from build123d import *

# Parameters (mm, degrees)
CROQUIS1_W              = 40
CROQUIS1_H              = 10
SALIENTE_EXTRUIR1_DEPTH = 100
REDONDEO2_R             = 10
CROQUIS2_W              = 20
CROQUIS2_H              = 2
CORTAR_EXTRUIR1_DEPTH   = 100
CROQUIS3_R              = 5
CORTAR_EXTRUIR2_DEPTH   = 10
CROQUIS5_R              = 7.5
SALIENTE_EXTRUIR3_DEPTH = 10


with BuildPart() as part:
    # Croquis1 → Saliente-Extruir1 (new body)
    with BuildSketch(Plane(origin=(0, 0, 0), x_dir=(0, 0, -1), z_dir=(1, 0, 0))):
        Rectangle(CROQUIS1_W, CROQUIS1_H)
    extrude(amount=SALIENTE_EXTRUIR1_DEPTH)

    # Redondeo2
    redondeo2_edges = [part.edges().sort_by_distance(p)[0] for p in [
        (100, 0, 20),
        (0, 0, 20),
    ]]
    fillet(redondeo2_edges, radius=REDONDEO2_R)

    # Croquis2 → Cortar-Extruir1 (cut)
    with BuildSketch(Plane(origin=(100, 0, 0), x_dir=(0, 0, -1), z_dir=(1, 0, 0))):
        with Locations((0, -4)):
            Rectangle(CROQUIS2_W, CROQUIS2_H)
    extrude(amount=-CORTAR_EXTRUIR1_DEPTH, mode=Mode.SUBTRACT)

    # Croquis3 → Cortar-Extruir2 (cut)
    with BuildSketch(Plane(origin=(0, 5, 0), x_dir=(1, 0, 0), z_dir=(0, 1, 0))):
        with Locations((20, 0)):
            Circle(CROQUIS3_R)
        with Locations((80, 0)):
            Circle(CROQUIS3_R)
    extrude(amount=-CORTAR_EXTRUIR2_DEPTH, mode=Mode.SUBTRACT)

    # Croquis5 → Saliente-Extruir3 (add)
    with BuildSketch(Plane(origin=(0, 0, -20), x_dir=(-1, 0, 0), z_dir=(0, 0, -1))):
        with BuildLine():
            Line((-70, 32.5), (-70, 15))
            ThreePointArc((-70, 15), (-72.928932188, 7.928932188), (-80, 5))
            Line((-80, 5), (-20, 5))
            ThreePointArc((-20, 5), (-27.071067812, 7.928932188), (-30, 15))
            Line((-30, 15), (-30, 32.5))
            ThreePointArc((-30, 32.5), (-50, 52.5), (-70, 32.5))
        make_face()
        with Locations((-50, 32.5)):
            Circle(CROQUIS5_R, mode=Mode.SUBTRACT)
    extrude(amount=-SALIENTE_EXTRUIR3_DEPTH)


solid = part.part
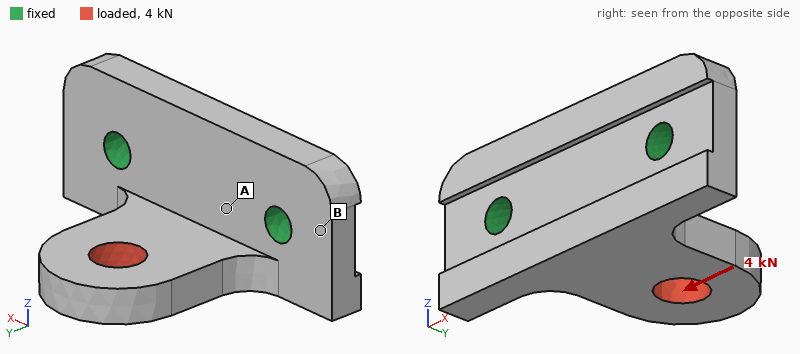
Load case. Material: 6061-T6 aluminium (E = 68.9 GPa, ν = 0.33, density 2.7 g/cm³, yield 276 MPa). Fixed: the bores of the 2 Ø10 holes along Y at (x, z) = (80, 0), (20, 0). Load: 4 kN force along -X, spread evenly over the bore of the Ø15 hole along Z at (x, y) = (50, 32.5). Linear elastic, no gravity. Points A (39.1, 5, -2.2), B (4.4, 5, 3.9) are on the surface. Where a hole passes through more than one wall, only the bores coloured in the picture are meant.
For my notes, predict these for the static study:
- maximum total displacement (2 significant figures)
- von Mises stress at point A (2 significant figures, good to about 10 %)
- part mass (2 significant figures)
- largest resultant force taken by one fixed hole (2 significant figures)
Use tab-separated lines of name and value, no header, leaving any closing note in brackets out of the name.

maximum total displacement	83 µm
von Mises stress at point A	23 MPa
part mass	140 g
largest resultant force taken by one fixed hole	3.2 kN
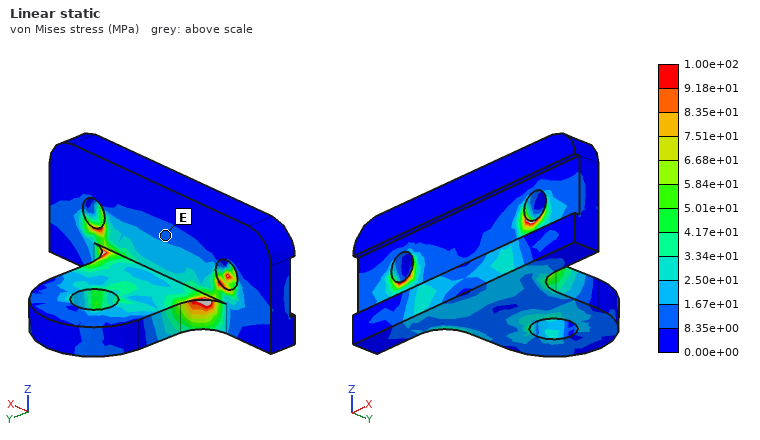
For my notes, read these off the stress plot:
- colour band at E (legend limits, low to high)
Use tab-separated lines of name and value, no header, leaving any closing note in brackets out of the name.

colour band at E	8.35e+00 to 1.67e+01 MPa
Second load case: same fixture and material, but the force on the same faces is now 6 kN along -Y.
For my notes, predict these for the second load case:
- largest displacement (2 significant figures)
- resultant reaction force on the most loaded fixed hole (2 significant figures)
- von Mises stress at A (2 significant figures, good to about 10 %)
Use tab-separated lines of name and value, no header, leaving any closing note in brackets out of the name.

largest displacement	0.16 mm
resultant reaction force on the most loaded fixed hole	3.1 kN
von Mises stress at A	29 MPa
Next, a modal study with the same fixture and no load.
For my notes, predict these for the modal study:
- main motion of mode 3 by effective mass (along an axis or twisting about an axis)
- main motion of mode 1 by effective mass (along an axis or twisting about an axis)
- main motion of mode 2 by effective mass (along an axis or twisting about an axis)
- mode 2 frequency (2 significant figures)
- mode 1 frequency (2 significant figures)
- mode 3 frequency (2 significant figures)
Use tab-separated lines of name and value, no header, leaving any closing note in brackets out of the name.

main motion of mode 3 by effective mass	along Y
main motion of mode 1 by effective mass	along Z
main motion of mode 2 by effective mass	along X
mode 2 frequency	6900 Hz
mode 1 frequency	2600 Hz
mode 3 frequency	8300 Hz
